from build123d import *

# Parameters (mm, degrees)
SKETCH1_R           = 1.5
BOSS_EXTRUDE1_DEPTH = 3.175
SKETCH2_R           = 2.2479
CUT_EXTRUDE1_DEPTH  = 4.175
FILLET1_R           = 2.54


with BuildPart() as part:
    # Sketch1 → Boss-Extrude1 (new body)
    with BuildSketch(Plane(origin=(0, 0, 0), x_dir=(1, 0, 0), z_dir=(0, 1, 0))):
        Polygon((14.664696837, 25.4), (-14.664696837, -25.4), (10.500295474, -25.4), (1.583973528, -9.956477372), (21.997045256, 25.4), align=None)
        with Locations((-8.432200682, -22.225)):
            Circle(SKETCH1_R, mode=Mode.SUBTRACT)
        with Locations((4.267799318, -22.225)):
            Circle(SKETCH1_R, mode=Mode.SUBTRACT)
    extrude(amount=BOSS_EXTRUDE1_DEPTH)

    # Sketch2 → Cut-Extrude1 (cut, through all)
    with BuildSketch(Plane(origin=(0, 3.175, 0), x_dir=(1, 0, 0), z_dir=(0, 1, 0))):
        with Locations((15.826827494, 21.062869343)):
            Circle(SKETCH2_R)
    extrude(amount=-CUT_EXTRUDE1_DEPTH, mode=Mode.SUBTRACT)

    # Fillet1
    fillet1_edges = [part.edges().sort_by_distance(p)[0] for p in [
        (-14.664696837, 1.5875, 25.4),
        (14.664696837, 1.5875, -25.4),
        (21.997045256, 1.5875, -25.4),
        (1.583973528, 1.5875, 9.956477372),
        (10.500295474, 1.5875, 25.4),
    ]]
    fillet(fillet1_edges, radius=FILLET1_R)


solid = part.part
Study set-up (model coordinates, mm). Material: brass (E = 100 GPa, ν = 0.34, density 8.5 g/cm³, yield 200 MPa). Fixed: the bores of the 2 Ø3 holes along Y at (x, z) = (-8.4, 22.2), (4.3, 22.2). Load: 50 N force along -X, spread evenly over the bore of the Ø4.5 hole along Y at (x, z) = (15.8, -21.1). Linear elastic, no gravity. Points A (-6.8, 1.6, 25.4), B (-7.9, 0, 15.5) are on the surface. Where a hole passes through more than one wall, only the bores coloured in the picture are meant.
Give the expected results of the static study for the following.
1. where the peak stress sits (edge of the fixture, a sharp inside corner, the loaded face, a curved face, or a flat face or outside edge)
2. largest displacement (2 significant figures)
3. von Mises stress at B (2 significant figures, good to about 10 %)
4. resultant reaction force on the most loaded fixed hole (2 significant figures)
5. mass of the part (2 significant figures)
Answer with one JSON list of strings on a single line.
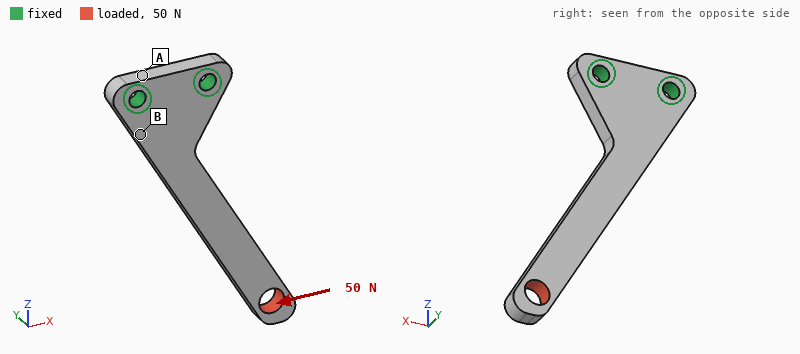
["a curved face", "0.14 mm", "16 MPa", "160 N", "13 g"]
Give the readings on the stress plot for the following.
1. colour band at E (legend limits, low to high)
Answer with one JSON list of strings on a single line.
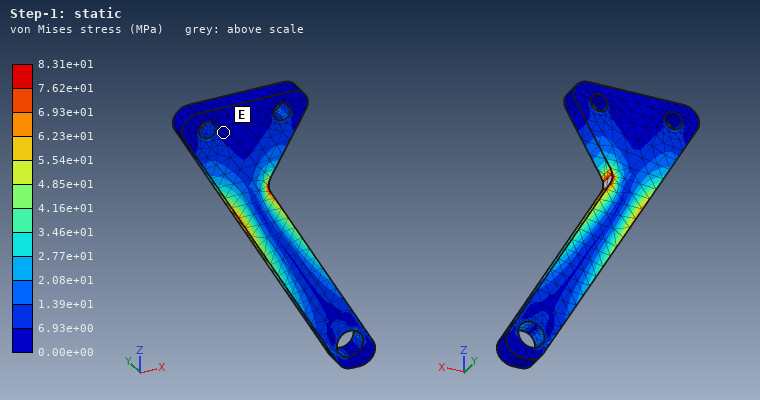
["0.00e+00 to 6.93e+00 MPa"]
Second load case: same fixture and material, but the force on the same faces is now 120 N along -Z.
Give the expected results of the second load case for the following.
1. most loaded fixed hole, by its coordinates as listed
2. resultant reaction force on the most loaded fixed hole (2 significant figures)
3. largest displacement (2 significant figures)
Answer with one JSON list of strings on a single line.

["(4.3, 22.2)", "220 N", "0.19 mm"]
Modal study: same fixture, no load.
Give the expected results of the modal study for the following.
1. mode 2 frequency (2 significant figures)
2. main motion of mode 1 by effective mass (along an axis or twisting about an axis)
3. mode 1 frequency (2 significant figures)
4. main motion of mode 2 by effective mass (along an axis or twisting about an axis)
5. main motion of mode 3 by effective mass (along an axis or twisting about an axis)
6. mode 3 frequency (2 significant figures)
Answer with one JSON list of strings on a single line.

["2100 Hz", "along Y", "890 Hz", "along X", "along Y", "4700 Hz"]
